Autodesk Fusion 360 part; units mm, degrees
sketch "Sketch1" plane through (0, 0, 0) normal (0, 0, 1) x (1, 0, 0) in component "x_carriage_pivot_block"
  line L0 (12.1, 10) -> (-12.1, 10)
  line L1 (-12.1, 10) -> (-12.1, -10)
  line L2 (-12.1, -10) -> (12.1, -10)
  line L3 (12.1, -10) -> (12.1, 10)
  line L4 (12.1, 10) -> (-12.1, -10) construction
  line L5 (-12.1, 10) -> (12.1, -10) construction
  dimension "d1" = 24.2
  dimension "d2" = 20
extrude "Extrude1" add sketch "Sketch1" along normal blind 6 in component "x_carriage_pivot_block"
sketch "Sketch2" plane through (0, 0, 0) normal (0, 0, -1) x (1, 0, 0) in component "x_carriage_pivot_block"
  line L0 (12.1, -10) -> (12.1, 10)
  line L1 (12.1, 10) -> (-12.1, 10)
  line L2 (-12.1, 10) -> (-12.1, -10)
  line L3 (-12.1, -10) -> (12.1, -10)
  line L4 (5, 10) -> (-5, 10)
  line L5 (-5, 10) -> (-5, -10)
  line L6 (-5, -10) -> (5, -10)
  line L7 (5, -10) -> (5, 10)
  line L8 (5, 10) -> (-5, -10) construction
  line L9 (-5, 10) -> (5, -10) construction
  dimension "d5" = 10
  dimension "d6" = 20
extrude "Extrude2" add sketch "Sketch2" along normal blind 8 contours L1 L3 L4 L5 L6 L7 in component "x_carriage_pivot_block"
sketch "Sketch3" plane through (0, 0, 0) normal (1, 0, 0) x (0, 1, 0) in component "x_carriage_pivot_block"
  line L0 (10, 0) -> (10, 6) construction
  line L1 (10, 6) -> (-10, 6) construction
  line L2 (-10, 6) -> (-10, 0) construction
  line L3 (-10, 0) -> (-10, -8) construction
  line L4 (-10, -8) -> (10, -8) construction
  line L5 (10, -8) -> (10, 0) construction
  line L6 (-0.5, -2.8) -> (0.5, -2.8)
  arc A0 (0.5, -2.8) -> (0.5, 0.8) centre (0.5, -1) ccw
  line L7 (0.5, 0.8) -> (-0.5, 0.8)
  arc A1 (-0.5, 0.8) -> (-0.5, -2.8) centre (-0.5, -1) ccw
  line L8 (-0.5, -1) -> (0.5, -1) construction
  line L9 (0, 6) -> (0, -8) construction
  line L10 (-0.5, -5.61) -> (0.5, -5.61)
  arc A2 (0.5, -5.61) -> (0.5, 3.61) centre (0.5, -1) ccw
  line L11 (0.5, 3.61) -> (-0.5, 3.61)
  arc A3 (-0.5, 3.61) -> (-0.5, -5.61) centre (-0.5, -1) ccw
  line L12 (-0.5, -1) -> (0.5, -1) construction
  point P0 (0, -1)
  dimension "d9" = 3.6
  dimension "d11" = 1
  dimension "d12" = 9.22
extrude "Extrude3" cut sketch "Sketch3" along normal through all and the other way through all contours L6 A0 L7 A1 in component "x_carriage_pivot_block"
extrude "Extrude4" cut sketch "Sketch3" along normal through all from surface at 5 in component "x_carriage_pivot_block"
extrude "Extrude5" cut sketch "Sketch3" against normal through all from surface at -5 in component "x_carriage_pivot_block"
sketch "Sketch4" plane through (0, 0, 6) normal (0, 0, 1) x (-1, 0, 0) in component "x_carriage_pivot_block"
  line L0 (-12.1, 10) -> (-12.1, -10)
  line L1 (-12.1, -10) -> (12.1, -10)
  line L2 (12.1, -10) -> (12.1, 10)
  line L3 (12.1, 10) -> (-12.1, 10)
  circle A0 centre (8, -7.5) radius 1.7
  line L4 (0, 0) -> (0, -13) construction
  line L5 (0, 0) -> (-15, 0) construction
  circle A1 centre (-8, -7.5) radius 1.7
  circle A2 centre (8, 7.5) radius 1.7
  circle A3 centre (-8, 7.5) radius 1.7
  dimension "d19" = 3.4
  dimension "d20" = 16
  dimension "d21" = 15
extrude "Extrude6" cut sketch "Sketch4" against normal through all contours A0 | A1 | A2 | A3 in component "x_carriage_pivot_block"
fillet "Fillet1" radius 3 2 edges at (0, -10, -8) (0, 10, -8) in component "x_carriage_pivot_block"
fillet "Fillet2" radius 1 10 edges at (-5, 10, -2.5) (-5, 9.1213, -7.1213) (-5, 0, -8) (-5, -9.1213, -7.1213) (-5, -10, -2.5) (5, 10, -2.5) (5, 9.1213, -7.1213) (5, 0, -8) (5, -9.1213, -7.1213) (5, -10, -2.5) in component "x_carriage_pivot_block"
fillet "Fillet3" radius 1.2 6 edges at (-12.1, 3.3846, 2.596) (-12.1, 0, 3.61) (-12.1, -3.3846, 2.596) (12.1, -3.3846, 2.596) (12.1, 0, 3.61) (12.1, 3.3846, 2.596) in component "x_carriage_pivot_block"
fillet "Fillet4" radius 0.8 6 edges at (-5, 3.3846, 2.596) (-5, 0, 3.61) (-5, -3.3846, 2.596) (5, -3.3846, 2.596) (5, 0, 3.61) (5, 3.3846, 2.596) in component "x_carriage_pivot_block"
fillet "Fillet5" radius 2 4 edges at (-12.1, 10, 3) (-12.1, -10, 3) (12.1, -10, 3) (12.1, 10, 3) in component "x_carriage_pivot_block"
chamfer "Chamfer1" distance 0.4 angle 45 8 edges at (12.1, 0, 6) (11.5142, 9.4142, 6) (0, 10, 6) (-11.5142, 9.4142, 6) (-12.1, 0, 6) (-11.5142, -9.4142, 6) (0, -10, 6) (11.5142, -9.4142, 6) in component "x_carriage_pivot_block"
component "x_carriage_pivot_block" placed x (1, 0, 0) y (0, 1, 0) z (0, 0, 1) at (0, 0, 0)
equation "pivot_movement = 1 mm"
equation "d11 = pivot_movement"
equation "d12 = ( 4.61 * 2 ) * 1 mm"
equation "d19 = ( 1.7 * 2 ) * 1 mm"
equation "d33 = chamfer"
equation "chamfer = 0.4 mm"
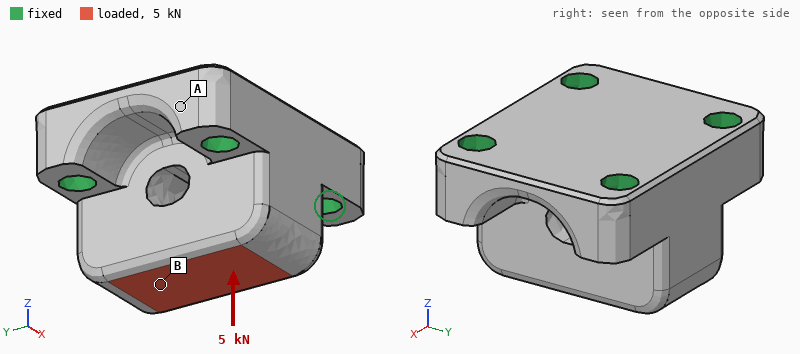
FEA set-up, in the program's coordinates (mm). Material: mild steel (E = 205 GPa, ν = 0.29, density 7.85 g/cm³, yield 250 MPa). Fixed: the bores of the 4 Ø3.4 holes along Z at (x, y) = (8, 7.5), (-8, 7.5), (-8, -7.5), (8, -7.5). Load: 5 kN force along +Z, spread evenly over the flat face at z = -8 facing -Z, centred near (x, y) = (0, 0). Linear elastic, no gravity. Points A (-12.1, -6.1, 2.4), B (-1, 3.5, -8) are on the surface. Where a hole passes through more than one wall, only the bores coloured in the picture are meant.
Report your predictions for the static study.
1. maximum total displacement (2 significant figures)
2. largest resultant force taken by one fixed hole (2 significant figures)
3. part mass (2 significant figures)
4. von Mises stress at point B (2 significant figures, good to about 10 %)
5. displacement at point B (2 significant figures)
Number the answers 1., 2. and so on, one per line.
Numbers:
1. 4.2 µm
2. 1.3 kN
3. 29 g
4. 23 MPa
5. 3.8 µm
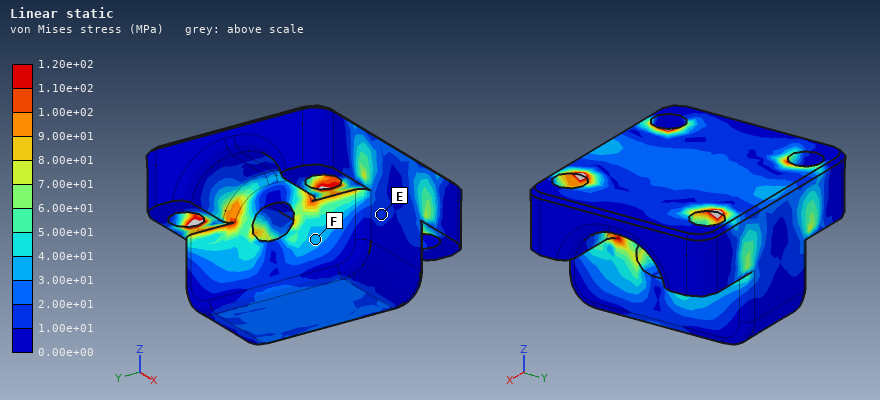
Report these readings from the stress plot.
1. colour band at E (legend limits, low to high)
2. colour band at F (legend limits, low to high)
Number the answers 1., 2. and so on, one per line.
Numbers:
1. 1.00e+01 to 2.00e+01 MPa
2. 3.00e+01 to 4.00e+01 MPa
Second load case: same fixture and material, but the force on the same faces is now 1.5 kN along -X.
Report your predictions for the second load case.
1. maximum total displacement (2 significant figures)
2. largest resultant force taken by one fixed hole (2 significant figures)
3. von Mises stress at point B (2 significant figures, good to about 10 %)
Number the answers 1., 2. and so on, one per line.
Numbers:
1. 4.8 µm
2. 730 N
3. 28 MPa
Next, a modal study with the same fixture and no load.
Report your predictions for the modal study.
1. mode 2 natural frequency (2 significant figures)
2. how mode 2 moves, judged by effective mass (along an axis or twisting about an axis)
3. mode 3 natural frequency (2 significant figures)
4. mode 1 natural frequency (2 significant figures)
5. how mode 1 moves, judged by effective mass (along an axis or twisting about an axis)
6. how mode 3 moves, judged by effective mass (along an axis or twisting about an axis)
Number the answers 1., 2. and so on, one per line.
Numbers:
1. 43 kHz
2. along X
3. 54 kHz
4. 39 kHz
5. along Y
6. along Z
